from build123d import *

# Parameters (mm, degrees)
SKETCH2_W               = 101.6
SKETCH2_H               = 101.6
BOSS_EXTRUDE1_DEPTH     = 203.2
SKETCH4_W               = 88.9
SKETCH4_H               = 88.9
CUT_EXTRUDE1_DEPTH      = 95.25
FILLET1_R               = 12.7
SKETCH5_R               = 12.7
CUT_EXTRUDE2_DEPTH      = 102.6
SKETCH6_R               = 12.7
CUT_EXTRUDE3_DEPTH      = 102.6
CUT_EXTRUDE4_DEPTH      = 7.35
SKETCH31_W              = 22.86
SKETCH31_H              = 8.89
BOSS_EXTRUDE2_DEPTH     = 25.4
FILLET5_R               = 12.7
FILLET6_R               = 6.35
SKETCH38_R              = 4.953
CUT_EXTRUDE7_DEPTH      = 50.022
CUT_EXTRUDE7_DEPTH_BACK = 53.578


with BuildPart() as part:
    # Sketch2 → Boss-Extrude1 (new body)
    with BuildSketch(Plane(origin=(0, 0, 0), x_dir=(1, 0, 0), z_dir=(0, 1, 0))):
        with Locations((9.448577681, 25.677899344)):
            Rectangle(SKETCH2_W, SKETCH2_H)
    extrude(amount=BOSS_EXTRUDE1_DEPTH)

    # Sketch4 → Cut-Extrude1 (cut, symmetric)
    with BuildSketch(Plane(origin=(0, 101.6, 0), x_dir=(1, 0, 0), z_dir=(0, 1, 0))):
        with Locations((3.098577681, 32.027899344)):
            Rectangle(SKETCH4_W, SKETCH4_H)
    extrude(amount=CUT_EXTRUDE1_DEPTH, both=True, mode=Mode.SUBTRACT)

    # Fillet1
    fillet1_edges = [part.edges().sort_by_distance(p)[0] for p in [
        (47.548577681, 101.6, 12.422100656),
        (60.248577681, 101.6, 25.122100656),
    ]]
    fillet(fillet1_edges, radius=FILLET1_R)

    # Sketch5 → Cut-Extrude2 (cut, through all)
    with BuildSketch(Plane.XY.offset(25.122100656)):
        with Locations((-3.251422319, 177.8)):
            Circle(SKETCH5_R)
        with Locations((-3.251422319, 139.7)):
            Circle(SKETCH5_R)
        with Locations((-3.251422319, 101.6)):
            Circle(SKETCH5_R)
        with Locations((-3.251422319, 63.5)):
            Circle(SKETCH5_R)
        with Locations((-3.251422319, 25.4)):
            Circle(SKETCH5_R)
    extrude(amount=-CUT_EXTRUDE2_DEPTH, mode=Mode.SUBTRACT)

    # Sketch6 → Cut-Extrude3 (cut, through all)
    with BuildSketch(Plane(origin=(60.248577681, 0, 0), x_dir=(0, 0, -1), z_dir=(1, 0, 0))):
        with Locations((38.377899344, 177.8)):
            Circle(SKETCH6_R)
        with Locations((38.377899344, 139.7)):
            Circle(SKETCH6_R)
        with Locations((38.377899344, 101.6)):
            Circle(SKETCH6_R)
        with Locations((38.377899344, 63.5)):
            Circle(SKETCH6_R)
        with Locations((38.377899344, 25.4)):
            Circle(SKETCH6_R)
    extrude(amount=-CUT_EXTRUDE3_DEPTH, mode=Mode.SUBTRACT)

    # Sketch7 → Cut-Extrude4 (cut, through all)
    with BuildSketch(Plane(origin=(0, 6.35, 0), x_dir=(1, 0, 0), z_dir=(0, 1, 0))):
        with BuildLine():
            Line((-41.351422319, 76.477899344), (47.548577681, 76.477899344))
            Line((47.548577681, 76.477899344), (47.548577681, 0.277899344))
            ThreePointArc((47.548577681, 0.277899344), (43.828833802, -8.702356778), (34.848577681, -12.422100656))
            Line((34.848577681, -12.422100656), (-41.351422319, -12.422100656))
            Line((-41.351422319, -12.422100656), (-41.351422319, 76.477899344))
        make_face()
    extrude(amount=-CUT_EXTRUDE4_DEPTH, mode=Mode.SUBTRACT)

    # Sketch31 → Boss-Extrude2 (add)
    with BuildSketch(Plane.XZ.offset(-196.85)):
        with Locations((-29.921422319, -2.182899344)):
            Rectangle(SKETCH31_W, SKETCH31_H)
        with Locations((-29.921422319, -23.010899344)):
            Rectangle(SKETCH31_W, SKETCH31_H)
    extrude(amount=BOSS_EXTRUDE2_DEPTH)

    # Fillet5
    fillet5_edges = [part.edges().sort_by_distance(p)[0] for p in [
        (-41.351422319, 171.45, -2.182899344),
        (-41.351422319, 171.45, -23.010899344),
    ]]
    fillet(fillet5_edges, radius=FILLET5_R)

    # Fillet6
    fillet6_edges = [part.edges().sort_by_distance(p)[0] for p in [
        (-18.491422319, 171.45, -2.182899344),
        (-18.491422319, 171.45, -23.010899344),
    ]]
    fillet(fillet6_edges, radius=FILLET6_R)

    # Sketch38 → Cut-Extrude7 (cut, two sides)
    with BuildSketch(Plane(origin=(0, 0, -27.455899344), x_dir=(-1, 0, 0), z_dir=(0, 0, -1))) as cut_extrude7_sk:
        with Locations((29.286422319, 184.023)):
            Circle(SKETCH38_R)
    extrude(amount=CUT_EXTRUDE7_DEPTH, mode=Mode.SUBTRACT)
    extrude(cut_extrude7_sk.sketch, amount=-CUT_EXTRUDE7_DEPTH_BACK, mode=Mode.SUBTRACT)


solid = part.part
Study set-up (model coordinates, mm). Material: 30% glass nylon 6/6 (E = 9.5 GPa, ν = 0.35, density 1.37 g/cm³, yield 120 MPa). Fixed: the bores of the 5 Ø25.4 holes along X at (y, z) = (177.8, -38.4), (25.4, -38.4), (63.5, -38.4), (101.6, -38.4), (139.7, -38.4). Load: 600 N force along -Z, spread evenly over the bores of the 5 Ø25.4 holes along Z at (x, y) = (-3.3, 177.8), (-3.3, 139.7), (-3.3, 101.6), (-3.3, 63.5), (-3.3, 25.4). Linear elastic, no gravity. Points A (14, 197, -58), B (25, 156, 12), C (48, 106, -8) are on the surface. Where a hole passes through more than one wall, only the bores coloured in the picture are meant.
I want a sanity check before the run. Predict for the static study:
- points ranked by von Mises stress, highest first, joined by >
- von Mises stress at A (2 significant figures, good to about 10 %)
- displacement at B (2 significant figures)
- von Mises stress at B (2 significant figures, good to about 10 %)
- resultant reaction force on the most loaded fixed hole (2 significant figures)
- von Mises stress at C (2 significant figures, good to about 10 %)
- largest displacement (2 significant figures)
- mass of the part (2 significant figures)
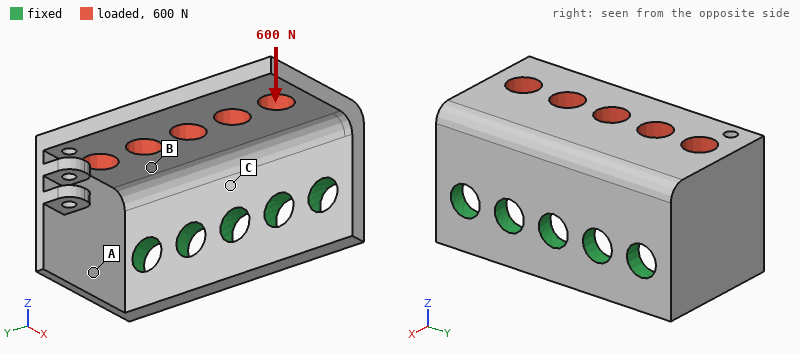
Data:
C > B > A
0.67 MPa
0.076 mm
2.3 MPa
160 N
4.2 MPa
0.44 mm
660 g
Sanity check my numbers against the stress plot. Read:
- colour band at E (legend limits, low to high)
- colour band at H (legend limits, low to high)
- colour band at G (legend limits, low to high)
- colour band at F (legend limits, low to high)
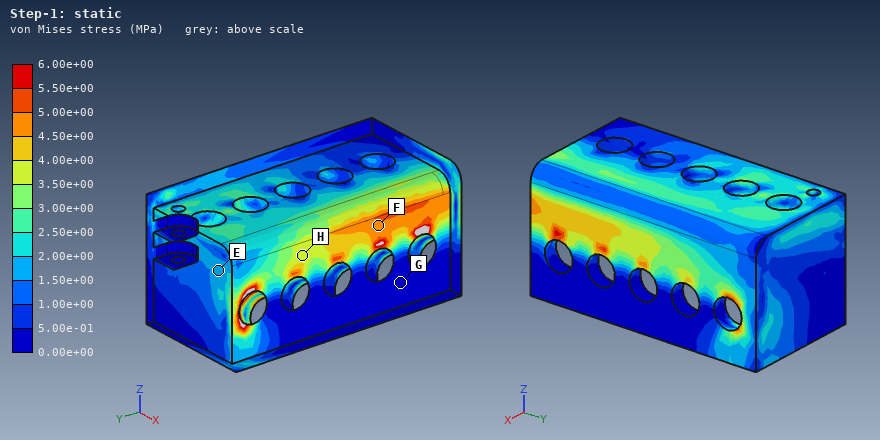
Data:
1.50e+00 to 2.00e+00 MPa
3.50e+00 to 4.00e+00 MPa
0.00e+00 to 5.00e-01 MPa
4.50e+00 to 5.00e+00 MPa
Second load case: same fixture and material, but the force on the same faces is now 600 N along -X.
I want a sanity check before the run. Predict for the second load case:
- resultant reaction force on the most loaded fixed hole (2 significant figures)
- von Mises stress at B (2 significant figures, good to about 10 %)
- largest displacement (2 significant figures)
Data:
140 N
0.79 MPa
0.17 mm
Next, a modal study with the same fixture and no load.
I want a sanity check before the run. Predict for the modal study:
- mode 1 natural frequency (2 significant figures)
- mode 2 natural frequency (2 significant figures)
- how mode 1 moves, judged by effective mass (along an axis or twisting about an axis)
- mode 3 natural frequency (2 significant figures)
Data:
450 Hz
600 Hz
along Z
710 Hz
